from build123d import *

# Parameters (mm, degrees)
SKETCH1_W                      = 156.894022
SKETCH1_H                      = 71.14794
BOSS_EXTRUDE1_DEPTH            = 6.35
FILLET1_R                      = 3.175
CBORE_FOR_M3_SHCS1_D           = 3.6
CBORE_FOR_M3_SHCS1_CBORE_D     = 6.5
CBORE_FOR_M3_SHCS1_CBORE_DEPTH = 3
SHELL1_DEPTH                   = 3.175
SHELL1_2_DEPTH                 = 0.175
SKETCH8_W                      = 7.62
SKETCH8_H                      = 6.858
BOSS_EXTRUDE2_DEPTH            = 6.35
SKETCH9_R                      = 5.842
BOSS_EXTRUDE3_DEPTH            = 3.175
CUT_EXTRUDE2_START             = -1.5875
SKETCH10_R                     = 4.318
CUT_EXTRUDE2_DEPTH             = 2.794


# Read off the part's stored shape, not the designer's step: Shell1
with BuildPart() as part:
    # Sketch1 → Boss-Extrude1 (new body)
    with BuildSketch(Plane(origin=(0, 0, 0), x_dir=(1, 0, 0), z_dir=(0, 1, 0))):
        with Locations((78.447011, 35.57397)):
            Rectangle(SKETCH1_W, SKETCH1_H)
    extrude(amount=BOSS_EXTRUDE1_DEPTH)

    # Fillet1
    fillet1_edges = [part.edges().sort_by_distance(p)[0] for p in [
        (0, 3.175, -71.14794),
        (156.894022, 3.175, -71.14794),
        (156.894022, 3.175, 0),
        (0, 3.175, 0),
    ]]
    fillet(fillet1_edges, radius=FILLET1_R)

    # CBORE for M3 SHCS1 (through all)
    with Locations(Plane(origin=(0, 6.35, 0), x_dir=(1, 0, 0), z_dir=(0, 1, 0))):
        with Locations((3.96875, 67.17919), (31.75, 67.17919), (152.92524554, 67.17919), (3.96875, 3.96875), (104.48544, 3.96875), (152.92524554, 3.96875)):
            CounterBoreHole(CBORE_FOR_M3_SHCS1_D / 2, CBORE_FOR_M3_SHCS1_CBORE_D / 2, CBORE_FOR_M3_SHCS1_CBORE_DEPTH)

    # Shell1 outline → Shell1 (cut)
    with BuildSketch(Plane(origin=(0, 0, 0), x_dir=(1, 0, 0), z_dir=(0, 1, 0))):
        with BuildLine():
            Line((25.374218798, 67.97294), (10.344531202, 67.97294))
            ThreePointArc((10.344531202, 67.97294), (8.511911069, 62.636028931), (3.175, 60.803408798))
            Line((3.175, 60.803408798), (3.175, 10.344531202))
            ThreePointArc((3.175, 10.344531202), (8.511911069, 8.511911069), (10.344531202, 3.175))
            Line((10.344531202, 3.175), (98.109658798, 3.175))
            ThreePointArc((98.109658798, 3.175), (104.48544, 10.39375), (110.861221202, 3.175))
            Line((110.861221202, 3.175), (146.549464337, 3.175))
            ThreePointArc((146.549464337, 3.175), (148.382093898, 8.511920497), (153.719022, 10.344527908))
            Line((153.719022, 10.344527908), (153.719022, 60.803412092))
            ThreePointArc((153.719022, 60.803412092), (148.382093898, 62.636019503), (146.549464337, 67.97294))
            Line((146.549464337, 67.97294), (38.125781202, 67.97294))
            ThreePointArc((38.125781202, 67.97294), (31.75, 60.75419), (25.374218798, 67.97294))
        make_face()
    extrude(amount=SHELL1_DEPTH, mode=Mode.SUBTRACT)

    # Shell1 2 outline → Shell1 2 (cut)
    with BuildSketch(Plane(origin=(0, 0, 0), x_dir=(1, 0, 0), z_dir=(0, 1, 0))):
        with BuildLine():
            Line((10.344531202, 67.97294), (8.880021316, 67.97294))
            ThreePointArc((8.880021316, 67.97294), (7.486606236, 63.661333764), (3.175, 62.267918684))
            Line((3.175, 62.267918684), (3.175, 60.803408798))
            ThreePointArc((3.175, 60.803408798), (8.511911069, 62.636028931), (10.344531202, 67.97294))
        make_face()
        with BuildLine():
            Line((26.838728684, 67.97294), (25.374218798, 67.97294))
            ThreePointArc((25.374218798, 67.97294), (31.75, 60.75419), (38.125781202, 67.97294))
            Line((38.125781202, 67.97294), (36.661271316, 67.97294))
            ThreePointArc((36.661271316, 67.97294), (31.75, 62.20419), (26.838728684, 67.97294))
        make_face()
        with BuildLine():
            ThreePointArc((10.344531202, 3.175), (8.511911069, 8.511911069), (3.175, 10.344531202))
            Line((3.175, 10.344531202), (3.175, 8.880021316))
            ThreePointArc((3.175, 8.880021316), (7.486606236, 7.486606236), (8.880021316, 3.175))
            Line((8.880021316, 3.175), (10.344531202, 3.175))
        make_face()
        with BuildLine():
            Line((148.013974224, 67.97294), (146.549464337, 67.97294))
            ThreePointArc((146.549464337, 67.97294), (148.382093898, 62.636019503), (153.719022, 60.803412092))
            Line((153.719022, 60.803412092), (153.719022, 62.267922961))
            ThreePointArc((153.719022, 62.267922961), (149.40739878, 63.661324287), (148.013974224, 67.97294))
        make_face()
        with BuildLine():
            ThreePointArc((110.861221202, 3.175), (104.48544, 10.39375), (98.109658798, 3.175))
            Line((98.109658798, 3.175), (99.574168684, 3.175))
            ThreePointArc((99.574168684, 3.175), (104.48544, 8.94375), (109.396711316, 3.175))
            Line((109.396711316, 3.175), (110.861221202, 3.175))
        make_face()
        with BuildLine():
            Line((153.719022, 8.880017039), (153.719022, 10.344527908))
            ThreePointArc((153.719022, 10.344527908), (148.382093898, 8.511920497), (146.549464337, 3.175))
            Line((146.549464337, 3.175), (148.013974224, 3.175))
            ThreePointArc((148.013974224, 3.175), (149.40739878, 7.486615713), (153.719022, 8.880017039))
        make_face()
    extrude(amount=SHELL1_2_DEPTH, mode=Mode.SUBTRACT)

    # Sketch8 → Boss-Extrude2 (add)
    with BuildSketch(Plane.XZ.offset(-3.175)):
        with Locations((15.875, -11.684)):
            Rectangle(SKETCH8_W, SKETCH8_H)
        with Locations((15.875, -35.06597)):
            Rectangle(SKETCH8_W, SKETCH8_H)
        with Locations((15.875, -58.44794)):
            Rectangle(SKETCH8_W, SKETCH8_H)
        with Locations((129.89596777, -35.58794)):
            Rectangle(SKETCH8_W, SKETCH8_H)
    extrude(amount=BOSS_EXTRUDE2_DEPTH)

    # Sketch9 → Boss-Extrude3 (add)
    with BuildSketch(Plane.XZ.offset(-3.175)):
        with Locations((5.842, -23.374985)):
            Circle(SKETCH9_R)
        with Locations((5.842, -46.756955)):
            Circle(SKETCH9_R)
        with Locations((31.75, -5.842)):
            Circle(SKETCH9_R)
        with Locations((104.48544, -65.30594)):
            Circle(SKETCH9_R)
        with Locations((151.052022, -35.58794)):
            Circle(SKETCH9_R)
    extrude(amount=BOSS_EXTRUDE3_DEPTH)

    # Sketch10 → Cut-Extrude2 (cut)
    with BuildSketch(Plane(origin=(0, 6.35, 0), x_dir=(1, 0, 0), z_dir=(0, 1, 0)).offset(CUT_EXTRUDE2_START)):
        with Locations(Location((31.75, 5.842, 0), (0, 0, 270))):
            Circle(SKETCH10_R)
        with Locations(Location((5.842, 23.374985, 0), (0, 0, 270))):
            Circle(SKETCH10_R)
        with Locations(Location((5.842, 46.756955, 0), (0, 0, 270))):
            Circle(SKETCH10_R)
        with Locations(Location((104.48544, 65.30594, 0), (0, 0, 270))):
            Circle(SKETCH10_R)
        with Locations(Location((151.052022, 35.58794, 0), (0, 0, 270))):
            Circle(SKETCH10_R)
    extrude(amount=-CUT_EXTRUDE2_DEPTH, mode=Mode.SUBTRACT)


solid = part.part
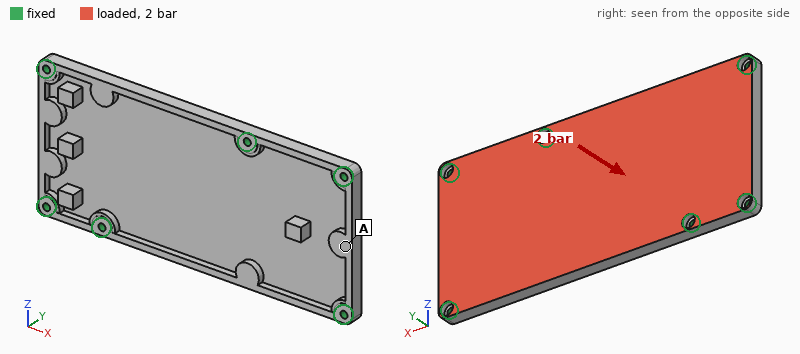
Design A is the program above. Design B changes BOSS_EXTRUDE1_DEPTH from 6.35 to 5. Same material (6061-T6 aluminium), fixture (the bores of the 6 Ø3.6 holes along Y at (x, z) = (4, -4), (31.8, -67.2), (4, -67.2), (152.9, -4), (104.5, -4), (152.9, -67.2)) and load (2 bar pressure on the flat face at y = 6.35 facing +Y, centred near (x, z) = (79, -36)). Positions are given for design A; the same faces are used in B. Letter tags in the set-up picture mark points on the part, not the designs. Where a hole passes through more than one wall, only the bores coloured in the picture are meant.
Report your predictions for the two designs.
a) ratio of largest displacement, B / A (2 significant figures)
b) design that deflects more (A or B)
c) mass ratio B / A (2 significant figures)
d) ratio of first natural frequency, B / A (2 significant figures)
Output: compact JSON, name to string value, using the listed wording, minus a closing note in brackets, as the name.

{"ratio of largest displacement, B / A": "3.0", "design that deflects more": "B", "mass ratio B / A": "0.65", "ratio of first natural frequency, B / A": "0.76"}
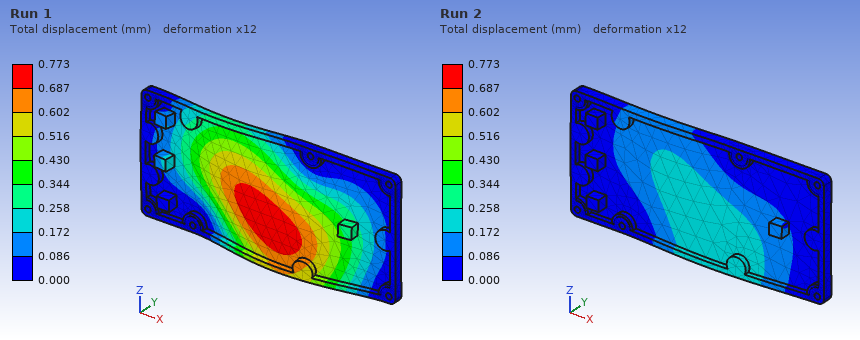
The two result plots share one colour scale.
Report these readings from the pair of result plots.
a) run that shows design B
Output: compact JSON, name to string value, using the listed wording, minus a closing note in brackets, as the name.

{"run that shows design B": "Run 1"}
